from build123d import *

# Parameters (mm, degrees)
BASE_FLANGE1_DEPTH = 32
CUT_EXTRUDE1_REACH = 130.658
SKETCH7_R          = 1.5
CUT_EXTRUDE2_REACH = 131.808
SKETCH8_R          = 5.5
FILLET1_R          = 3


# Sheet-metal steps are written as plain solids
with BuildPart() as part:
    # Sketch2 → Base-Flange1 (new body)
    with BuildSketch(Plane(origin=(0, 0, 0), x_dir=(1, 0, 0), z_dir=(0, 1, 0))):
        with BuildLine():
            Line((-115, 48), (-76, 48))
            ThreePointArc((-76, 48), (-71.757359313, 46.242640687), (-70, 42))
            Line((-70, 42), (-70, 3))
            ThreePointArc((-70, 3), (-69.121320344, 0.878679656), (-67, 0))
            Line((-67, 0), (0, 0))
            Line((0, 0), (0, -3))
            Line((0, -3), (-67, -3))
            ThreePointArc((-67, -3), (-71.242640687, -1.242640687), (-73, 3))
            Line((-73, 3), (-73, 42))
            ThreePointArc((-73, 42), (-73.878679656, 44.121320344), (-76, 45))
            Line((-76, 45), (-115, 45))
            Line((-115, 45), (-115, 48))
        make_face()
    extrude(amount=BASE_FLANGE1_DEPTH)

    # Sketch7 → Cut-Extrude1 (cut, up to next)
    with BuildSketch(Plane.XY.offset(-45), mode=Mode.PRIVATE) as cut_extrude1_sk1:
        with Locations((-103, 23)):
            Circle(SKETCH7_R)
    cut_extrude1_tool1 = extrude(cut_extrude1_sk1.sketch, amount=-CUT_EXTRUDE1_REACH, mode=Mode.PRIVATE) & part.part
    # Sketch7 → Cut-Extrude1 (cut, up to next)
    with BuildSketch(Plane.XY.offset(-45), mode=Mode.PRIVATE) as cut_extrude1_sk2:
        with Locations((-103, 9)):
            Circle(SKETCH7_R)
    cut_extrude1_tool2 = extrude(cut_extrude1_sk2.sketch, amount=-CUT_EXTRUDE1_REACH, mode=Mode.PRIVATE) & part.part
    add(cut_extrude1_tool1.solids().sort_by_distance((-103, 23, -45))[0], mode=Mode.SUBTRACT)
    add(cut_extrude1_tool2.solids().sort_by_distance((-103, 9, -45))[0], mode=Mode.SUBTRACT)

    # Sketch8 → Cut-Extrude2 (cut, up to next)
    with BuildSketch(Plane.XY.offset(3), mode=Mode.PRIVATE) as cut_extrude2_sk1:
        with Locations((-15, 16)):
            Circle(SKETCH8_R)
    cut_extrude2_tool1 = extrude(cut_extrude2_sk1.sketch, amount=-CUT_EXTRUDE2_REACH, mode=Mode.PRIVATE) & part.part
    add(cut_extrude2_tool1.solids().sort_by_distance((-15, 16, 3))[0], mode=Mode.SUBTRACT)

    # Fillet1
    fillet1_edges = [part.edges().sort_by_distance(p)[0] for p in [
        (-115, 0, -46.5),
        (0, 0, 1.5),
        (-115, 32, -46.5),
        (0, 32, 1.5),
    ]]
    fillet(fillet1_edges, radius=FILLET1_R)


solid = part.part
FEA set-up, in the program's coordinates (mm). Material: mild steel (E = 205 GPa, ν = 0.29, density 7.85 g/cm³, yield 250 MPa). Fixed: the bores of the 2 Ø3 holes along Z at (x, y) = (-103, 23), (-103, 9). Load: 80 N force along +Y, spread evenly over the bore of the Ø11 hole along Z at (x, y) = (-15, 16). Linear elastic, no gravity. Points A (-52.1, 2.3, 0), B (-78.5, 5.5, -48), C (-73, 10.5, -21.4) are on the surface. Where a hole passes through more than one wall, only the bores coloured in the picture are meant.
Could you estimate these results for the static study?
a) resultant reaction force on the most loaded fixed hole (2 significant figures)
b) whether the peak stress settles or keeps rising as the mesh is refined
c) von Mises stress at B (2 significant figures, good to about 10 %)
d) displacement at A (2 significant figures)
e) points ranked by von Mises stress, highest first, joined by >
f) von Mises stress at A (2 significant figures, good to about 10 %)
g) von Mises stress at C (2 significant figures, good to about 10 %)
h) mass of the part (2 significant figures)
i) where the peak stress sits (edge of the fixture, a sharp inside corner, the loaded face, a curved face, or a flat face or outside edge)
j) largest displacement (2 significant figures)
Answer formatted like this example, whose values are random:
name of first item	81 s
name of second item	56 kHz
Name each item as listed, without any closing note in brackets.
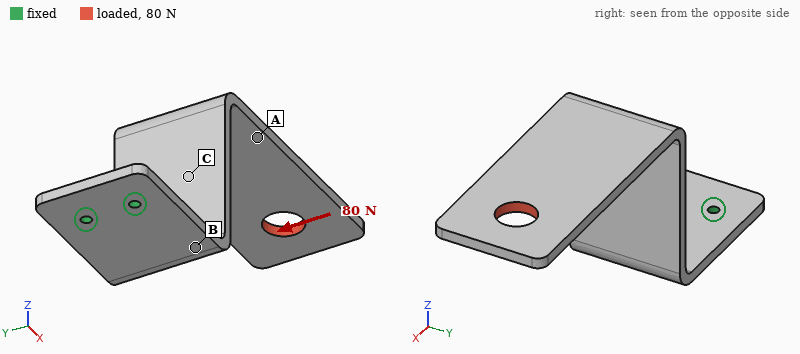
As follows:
resultant reaction force on the most loaded fixed hole	490 N
whether the peak stress settles or keeps rising as the mesh is refined	keeps rising
von Mises stress at B	43 MPa
displacement at A	0.31 mm
points ranked by von Mises stress, highest first, joined by >	C > B > A
von Mises stress at A	12 MPa
von Mises stress at C	79 MPa
mass of the part	120 g
where the peak stress sits	edge of the fixture
largest displacement	0.70 mm
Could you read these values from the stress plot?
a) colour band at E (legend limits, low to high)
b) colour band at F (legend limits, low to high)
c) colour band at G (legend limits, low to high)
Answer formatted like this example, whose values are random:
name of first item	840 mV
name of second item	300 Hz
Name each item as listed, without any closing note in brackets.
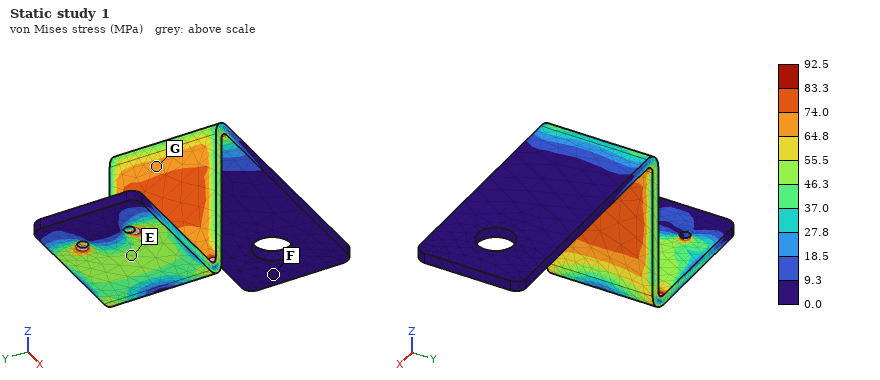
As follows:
colour band at E	46.3 to 55.5 MPa
colour band at F	0.0 to 9.3 MPa
colour band at G	64.8 to 74.0 MPa
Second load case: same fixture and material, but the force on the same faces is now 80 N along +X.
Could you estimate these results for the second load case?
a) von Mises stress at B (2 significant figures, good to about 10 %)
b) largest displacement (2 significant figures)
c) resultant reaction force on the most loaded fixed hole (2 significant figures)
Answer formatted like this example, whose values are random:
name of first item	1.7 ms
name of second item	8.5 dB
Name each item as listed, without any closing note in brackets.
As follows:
von Mises stress at B	73 MPa
largest displacement	1.2 mm
resultant reaction force on the most loaded fixed hole	41 N
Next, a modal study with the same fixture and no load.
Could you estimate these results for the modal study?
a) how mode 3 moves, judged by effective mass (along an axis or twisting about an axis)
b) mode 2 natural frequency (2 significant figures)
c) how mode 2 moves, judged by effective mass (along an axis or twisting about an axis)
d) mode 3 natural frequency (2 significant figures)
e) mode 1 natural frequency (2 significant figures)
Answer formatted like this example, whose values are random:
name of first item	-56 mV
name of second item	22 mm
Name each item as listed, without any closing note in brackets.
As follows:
how mode 3 moves, judged by effective mass	along X
mode 2 natural frequency	330 Hz
how mode 2 moves, judged by effective mass	along Y
mode 3 natural frequency	600 Hz
mode 1 natural frequency	160 Hz
